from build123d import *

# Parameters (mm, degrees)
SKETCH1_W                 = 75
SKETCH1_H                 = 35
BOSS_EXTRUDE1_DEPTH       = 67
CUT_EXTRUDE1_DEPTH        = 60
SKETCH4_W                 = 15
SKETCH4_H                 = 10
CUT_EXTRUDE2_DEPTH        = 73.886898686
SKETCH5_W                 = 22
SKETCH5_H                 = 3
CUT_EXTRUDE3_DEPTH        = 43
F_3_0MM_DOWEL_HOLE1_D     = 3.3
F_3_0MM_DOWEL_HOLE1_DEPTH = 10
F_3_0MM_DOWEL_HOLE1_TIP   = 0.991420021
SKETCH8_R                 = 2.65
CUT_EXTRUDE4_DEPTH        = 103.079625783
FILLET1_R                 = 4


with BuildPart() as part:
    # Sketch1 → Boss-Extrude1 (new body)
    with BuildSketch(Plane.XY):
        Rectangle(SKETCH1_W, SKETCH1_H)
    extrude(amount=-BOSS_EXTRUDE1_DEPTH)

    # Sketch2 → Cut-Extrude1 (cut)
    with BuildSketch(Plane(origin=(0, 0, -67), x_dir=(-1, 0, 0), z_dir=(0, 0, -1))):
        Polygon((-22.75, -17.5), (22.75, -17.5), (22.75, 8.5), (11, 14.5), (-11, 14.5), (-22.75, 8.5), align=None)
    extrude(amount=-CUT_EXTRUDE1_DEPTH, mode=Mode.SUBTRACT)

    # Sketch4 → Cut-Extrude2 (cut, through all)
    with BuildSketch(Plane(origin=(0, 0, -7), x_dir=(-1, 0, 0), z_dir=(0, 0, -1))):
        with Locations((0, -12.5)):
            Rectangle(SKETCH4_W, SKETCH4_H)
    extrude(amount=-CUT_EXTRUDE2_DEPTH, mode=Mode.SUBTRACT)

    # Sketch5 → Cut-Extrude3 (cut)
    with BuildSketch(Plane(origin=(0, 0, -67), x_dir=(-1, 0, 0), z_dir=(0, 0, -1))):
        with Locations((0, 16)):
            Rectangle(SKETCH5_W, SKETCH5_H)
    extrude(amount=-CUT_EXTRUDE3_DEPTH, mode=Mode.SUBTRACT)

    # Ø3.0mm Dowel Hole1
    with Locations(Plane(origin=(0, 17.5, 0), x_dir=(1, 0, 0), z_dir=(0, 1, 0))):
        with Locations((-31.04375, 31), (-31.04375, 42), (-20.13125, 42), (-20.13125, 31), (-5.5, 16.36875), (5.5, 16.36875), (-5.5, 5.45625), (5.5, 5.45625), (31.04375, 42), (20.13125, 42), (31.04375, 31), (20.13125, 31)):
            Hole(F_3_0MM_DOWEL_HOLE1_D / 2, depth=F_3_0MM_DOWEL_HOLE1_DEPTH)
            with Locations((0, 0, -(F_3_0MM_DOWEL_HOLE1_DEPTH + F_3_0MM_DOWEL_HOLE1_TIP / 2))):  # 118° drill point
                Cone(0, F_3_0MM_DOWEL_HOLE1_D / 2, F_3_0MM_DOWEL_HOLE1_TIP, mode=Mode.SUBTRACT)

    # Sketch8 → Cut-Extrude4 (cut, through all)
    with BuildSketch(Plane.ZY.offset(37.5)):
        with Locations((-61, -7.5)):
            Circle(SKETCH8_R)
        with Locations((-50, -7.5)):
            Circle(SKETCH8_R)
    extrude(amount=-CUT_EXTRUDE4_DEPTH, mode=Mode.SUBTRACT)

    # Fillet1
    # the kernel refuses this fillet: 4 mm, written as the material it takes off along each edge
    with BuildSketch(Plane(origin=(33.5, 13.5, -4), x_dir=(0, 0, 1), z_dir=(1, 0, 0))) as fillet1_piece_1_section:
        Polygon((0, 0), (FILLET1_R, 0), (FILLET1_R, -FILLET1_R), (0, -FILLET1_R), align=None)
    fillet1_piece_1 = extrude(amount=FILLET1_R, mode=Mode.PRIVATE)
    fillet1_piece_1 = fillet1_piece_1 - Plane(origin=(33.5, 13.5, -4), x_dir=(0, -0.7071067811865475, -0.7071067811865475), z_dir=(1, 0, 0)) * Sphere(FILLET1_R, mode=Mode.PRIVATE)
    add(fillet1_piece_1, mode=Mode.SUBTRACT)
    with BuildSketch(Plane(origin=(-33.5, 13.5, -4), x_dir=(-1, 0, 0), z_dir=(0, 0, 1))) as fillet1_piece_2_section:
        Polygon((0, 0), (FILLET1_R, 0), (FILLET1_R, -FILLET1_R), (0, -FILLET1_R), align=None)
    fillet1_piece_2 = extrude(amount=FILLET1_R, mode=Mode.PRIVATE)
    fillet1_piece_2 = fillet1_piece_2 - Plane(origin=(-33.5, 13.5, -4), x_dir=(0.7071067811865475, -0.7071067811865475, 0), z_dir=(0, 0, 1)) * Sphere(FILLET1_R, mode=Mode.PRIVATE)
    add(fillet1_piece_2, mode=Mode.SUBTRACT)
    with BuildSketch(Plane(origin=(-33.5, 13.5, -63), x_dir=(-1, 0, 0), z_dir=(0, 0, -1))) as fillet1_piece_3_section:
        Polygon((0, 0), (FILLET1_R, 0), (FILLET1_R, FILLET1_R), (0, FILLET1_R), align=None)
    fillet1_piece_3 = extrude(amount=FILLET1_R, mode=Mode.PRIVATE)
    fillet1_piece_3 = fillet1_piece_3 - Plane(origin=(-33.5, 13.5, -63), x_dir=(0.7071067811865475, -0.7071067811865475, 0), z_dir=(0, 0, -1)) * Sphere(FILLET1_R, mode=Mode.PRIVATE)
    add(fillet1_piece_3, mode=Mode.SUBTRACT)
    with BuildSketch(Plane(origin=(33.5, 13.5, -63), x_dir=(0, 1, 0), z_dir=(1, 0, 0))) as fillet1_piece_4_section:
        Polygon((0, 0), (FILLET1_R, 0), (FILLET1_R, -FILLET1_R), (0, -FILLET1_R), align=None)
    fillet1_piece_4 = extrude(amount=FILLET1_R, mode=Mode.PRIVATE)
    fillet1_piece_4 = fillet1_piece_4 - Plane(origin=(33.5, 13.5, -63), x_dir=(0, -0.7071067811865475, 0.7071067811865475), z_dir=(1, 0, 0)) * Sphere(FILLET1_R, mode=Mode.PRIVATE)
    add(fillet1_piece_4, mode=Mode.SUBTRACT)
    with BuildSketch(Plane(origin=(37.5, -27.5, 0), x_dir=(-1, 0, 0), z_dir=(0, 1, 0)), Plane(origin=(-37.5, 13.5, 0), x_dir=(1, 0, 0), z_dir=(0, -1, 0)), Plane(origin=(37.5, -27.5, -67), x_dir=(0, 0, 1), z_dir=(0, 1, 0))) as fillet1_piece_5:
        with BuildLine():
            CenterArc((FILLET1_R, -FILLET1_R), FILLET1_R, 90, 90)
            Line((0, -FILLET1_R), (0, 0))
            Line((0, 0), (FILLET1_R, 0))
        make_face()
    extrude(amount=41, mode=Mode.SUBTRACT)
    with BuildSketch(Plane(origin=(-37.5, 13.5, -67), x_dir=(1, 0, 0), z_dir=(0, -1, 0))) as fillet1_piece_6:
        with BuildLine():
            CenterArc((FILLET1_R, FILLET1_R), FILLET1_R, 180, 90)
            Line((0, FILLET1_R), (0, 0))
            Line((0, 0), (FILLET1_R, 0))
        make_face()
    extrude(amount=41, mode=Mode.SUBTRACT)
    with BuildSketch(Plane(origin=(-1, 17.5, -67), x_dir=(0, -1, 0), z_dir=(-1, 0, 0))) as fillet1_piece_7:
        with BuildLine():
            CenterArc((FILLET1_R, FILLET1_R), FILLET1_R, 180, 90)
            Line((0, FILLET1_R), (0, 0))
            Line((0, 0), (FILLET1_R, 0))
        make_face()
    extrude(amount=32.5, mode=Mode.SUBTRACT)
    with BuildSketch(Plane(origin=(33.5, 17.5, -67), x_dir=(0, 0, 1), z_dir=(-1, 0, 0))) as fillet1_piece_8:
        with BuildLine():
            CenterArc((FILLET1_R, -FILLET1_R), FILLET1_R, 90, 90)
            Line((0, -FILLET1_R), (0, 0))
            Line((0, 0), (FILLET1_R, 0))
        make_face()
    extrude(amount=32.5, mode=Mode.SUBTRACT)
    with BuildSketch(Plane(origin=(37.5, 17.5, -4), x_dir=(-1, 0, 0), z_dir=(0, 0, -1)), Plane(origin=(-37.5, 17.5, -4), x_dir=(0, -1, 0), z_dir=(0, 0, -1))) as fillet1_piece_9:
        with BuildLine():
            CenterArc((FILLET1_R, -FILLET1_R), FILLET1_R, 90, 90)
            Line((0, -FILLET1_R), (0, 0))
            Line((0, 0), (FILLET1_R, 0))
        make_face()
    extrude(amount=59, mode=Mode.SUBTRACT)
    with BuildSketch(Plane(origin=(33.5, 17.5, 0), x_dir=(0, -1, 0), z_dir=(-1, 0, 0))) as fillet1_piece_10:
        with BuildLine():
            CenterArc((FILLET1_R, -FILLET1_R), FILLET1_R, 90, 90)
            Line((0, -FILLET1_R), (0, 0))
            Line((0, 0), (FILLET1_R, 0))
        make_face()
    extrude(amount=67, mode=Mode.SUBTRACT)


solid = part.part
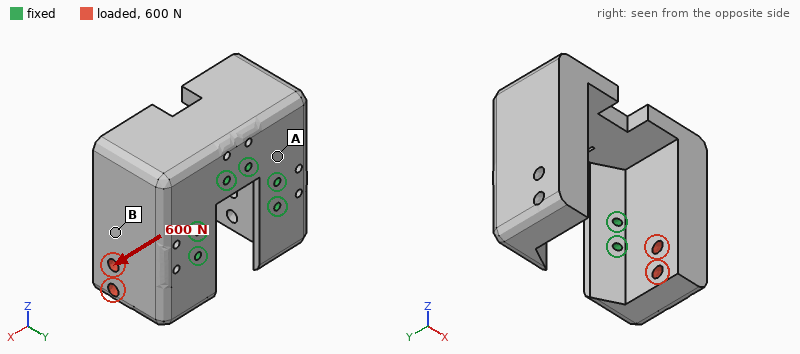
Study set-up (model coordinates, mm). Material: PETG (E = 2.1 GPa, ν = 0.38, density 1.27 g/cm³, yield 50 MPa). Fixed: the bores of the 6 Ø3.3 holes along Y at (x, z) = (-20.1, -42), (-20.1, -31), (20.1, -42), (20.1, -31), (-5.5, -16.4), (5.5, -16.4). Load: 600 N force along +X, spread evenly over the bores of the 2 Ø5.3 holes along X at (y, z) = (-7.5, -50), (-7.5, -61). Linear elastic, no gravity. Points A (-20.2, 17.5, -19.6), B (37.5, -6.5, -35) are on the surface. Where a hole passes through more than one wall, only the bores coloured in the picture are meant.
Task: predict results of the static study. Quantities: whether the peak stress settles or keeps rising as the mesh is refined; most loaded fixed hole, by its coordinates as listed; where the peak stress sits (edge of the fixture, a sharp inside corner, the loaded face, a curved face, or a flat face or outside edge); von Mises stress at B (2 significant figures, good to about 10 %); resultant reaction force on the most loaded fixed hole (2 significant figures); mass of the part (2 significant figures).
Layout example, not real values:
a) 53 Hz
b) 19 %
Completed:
a) keeps rising
b) (20.1, -42)
c) edge of the fixture
d) 6.6 MPa
e) 870 N
f) 110 g
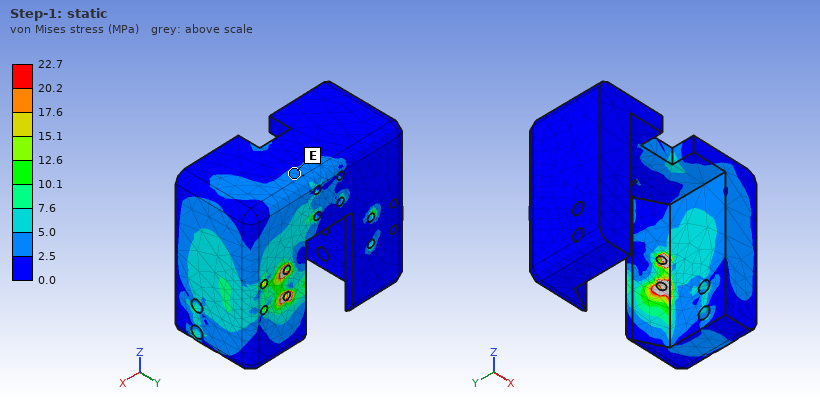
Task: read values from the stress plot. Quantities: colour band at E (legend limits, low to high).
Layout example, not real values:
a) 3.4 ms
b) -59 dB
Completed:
a) 2.5 to 5.0 MPa
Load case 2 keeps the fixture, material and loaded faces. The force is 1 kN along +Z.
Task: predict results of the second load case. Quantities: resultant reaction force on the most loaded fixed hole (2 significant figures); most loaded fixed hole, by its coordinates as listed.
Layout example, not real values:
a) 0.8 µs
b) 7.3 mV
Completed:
a) 1.1 kN
b) (20.1, -42)
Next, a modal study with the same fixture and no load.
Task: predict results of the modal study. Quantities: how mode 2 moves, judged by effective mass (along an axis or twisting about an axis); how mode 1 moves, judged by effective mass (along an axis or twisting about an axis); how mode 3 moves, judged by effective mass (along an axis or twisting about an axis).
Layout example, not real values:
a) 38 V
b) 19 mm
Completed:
a) along Z
b) along X
c) along Y
